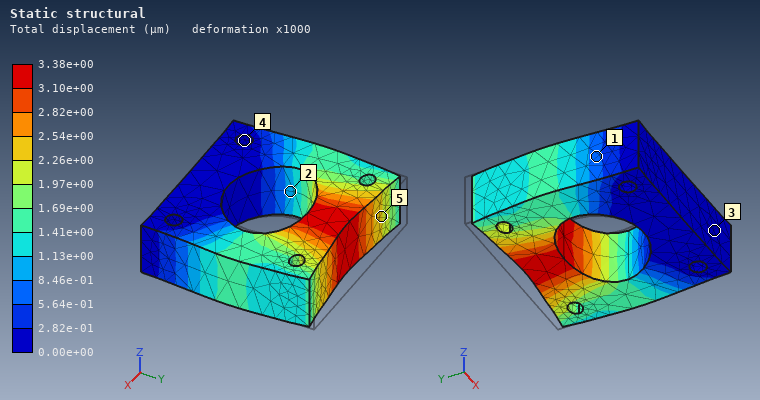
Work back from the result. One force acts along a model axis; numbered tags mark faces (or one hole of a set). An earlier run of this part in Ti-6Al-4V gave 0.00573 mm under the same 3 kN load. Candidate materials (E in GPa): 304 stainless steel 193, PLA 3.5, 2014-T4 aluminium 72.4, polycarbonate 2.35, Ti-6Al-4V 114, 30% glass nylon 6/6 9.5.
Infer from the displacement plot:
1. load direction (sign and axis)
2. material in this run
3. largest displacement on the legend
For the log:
-Y
304 stainless steel
3.38e+00 µm
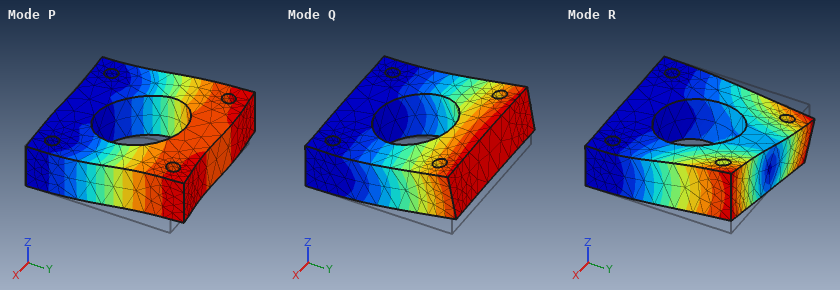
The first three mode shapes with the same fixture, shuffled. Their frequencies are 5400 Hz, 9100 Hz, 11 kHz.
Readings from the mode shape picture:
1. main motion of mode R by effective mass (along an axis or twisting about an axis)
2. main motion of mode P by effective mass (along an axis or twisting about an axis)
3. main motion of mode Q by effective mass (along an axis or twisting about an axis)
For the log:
twisting about Y
along X
along Z
